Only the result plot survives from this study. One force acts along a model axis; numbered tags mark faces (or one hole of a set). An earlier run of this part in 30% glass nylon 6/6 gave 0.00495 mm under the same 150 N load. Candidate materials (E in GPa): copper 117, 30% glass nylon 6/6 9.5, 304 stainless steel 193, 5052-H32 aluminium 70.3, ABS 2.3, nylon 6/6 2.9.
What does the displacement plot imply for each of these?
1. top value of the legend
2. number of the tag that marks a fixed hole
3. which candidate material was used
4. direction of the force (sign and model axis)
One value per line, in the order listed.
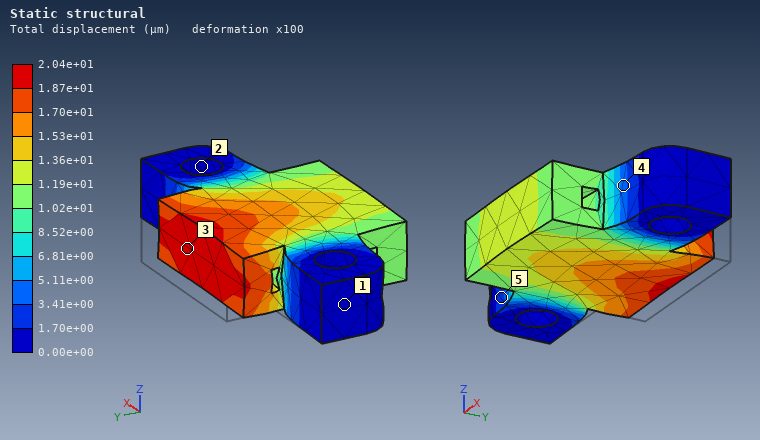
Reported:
2.04e+01 µm
2
ABS
-Y
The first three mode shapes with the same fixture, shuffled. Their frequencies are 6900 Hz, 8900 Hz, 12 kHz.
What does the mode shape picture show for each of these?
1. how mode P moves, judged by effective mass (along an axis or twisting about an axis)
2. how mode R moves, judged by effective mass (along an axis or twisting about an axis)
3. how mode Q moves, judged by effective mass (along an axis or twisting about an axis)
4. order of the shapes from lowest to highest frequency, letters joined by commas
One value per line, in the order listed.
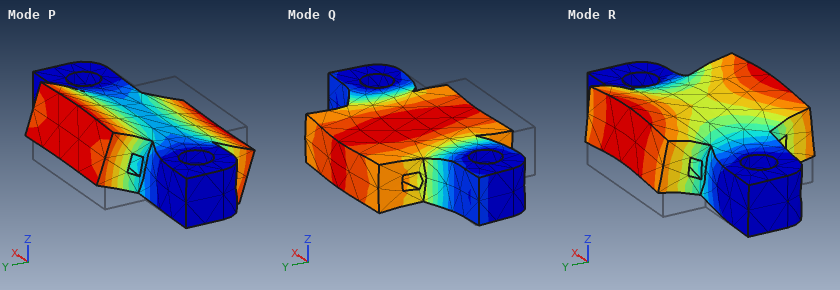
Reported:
twisting about X
along Z
along Y
P, R, Q
